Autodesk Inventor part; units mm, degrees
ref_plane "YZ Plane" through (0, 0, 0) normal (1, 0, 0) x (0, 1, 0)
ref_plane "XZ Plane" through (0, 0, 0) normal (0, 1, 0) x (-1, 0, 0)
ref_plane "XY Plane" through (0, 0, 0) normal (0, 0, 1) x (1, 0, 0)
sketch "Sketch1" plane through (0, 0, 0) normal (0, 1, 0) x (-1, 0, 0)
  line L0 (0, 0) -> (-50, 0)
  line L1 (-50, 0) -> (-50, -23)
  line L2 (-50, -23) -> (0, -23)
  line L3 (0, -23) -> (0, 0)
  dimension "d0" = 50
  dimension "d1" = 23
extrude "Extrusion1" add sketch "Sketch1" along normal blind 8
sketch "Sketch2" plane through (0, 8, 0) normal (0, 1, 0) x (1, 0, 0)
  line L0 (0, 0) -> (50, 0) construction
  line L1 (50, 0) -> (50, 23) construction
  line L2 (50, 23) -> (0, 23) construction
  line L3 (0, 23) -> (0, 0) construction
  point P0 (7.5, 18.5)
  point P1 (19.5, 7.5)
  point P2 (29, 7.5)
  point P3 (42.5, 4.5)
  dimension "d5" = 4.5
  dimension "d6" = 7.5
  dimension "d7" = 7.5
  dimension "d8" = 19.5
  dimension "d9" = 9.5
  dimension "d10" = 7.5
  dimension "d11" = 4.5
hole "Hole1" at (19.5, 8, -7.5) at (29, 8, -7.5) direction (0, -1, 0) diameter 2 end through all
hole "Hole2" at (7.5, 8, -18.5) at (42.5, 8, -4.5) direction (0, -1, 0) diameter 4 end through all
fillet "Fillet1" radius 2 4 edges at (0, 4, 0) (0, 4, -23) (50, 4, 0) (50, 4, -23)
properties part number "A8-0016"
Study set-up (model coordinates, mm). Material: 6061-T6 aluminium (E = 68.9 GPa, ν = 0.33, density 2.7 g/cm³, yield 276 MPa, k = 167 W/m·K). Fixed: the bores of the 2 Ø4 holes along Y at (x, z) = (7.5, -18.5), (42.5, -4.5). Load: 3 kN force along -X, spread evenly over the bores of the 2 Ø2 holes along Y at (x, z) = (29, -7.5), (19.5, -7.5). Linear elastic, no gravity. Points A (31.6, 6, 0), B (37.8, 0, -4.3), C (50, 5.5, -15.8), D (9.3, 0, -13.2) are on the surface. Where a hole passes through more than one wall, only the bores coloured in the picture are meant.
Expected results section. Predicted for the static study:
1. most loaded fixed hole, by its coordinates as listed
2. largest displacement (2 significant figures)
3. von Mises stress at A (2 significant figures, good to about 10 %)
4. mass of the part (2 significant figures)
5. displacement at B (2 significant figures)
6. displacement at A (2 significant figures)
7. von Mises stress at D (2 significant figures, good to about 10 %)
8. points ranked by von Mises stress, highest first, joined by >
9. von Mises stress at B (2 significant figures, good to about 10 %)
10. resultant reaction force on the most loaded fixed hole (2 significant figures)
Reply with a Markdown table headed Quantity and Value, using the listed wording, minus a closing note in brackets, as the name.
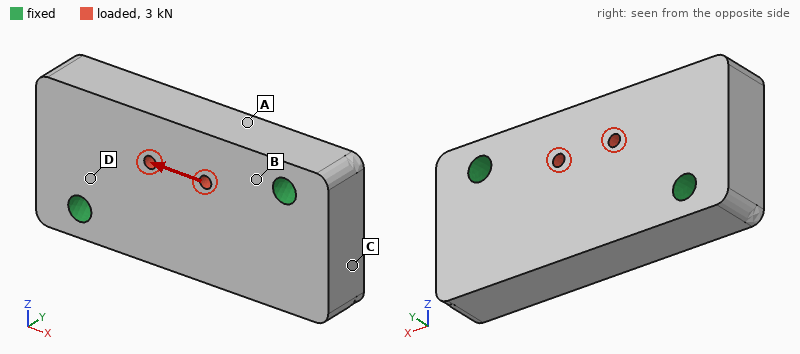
| Quantity | Value |
|---|---|
| most loaded fixed hole, by its coordinates as listed | (42.5, -4.5) |
| largest displacement | 6.3 µm |
| von Mises stress at A | 18 MPa |
| mass of the part | 24 g |
| displacement at B | 1.3 µm |
| displacement at A | 2.6 µm |
| von Mises stress at D | 11 MPa |
| points ranked by von Mises stress, highest first, joined by > | B > A > D > C |
| von Mises stress at B | 27 MPa |
| resultant reaction force on the most loaded fixed hole | 1.7 kN |
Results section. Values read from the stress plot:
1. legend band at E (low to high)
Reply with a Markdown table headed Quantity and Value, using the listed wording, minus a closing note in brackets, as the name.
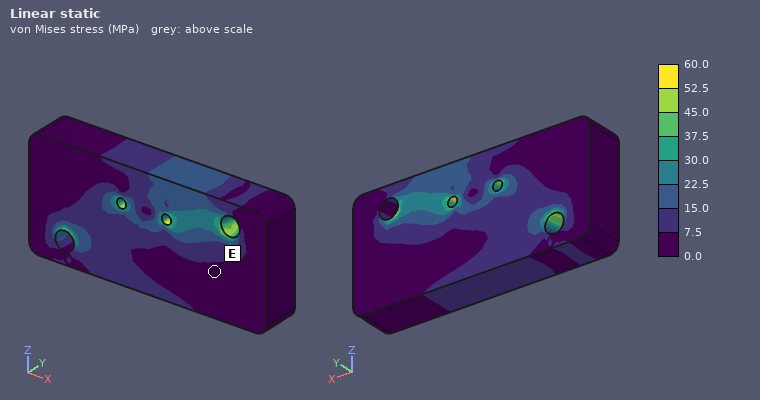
| Quantity | Value |
|---|---|
| legend band at E | 0.0 to 7.5 MPa |
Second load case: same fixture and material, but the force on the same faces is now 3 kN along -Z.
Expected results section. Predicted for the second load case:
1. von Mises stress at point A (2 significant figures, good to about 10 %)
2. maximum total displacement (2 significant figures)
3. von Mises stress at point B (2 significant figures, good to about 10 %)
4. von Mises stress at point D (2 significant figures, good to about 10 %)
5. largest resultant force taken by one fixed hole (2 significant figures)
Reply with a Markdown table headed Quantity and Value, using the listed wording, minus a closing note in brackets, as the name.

| Quantity | Value |
|---|---|
| von Mises stress at point A | 24 MPa |
| maximum total displacement | 10.0 µm |
| von Mises stress at point B | 23 MPa |
| von Mises stress at point D | 21 MPa |
| largest resultant force taken by one fixed hole | 1.6 kN |
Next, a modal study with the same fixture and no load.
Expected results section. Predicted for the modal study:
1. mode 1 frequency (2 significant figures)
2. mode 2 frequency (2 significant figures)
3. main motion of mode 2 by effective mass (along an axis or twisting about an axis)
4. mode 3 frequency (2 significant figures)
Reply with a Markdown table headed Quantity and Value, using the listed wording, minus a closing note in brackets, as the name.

| Quantity | Value |
|---|---|
| mode 1 frequency | 15 kHz |
| mode 2 frequency | 17 kHz |
| main motion of mode 2 by effective mass | along Y |
| mode 3 frequency | 25 kHz |
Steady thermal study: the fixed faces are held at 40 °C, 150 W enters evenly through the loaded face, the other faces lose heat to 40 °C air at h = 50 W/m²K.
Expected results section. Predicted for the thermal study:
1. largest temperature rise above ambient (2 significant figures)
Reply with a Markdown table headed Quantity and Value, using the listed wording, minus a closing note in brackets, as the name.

| Quantity | Value |
|---|---|
| largest temperature rise above ambient | 60 K |
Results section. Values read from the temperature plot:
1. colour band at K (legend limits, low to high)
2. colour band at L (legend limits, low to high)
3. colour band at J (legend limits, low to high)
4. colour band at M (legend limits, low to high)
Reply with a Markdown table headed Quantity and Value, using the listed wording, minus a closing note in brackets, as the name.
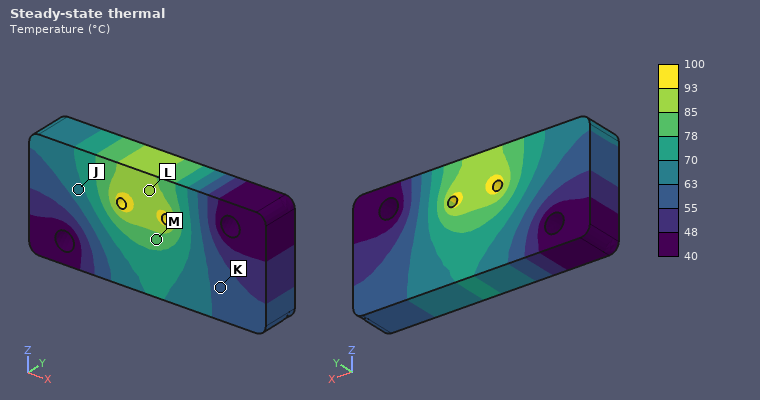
| Quantity | Value |
|---|---|
| colour band at K | 55 to 63 °C |
| colour band at L | 85 to 93 °C |
| colour band at J | 63 to 70 °C |
| colour band at M | 78 to 85 °C |
